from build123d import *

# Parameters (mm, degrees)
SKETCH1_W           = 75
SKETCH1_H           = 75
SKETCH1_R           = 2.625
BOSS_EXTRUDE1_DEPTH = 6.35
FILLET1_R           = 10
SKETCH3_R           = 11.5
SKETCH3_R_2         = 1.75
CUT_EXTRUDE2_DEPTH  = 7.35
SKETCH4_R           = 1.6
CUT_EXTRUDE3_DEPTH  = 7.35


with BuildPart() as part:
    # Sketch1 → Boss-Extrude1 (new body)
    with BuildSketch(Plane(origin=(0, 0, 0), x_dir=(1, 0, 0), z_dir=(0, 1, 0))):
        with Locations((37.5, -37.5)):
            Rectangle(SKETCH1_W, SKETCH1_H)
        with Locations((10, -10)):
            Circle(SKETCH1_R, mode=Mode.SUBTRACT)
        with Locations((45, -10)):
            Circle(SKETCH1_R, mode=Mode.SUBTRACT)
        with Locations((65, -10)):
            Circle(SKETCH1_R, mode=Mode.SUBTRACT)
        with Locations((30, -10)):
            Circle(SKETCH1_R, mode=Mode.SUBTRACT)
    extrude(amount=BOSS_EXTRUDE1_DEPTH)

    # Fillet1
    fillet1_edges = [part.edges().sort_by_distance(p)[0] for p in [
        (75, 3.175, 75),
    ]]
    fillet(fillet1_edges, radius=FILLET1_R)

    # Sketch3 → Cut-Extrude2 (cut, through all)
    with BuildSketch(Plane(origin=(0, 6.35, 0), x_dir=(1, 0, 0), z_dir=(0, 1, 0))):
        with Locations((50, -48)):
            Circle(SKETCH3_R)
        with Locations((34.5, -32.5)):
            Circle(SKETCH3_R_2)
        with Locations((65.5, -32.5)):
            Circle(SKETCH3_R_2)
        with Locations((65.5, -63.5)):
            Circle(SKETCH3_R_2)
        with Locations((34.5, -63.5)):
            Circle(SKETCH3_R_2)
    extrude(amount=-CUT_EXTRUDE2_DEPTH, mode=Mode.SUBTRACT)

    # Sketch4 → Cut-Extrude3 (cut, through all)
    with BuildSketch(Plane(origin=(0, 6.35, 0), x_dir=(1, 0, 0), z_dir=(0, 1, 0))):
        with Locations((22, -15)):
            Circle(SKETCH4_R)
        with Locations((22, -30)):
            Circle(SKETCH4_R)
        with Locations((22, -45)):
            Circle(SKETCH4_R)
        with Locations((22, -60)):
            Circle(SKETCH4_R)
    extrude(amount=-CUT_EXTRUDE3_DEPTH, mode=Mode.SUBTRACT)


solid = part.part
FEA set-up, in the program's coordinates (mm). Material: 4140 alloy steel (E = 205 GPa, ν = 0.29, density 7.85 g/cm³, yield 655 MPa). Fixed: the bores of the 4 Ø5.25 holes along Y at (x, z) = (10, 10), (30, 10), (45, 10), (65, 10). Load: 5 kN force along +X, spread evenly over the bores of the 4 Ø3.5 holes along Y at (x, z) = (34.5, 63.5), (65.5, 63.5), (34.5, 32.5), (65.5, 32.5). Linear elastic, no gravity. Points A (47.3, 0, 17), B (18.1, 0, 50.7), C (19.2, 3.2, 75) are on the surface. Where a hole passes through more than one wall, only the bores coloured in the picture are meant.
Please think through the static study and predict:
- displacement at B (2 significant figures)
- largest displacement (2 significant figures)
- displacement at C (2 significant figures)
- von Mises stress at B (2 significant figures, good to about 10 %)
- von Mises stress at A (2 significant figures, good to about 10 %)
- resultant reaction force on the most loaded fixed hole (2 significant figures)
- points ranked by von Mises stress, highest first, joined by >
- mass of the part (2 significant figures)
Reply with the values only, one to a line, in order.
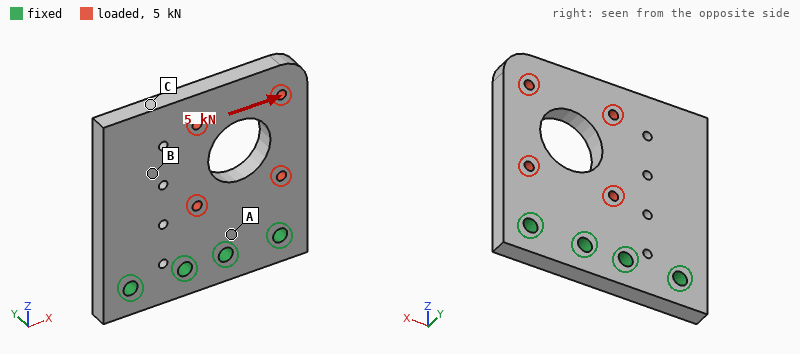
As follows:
9.3 µm
16 µm
15 µm
15 MPa
27 MPa
3.3 kN
A > B > C
250 g
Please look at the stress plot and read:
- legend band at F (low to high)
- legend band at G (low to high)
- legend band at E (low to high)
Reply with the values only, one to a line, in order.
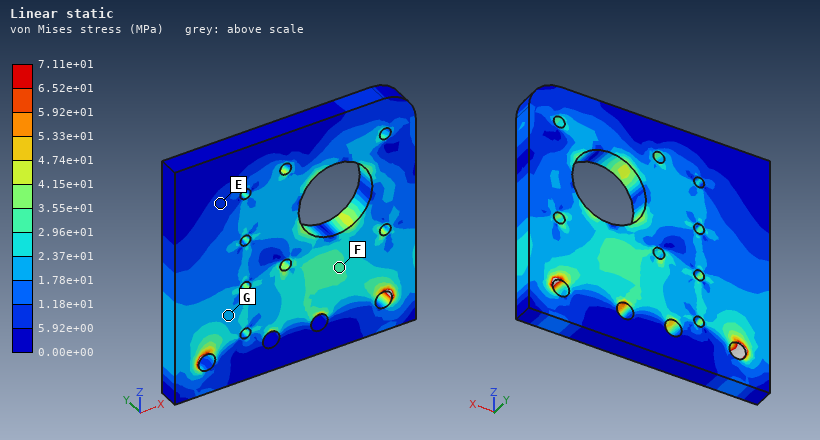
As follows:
2.96e+01 to 3.55e+01 MPa
1.78e+01 to 2.37e+01 MPa
5.92e+00 to 1.18e+01 MPa
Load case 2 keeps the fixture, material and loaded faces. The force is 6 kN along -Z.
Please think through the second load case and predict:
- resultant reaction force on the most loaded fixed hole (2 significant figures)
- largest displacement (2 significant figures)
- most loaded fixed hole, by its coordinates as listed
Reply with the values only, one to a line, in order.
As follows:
3.0 kN
7.2 µm
(65, 10)
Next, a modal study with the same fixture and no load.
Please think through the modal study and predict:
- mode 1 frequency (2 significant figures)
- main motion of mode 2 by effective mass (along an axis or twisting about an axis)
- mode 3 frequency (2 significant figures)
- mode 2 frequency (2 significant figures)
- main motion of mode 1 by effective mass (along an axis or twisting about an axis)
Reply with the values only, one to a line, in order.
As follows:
1300 Hz
twisting about Z
6500 Hz
2600 Hz
along Y
